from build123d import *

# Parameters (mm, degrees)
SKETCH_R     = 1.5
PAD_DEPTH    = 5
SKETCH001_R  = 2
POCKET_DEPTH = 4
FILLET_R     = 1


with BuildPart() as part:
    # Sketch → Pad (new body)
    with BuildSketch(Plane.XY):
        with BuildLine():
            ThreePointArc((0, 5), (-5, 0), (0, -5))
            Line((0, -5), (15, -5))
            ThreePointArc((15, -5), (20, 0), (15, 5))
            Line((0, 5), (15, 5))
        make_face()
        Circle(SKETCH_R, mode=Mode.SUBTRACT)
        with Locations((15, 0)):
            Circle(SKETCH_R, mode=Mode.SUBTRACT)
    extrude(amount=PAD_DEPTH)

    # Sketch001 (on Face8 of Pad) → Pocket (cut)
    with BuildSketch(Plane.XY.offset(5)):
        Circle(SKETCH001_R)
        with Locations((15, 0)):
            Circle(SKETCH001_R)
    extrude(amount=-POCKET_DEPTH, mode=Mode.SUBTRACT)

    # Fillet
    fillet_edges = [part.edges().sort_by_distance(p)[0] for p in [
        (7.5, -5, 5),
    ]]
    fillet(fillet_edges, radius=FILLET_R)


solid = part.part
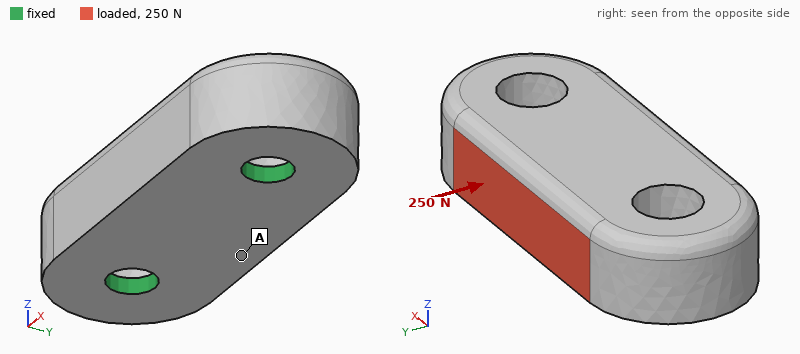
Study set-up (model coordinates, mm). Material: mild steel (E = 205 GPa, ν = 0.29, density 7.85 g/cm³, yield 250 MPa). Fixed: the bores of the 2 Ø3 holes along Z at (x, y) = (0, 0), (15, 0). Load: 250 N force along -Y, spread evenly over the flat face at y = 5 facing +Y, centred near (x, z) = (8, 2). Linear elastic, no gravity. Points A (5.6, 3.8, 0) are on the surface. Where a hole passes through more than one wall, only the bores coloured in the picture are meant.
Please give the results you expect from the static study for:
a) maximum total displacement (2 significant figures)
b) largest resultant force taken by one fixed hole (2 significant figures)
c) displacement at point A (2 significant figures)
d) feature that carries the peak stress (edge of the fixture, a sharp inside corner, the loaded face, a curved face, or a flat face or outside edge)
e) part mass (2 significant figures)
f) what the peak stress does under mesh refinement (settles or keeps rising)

1.5 µm
130 N
0.74 µm
edge of the fixture
8.0 g
keeps rising
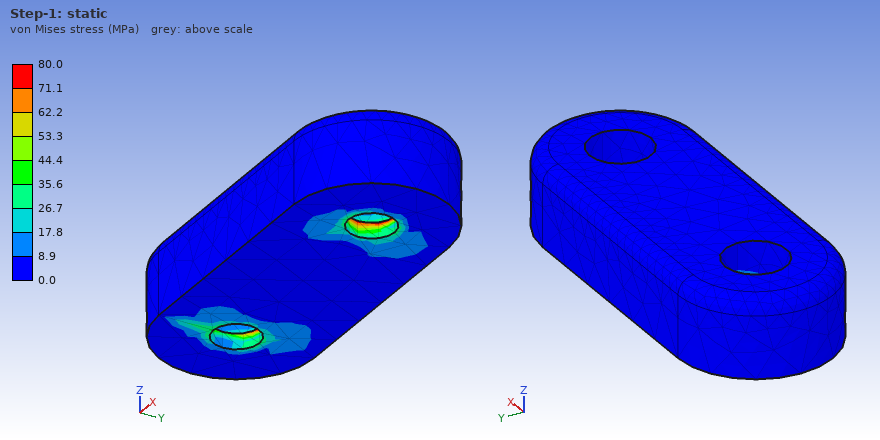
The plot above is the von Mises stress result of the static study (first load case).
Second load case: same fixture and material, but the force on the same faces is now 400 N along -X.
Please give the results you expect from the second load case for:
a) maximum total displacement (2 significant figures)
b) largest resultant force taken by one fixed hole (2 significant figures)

0.76 µm
230 N
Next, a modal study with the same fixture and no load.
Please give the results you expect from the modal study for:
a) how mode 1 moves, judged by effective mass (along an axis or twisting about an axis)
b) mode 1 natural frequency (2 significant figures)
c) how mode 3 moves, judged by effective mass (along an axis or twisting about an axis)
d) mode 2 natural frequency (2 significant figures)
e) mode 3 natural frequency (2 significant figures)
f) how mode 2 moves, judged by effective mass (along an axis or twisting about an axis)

along Y
22 kHz
twisting about Z
48 kHz
50 kHz
along Z
